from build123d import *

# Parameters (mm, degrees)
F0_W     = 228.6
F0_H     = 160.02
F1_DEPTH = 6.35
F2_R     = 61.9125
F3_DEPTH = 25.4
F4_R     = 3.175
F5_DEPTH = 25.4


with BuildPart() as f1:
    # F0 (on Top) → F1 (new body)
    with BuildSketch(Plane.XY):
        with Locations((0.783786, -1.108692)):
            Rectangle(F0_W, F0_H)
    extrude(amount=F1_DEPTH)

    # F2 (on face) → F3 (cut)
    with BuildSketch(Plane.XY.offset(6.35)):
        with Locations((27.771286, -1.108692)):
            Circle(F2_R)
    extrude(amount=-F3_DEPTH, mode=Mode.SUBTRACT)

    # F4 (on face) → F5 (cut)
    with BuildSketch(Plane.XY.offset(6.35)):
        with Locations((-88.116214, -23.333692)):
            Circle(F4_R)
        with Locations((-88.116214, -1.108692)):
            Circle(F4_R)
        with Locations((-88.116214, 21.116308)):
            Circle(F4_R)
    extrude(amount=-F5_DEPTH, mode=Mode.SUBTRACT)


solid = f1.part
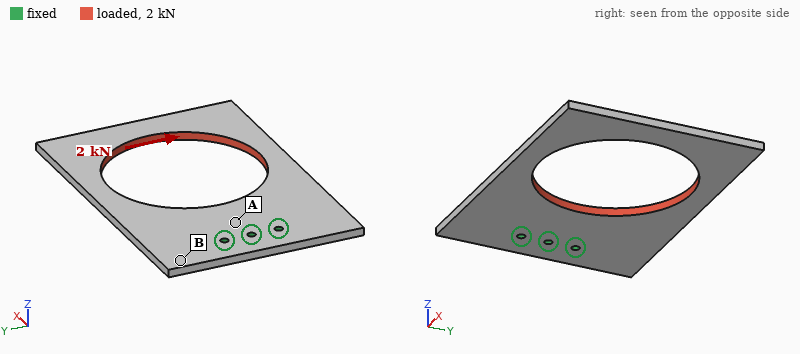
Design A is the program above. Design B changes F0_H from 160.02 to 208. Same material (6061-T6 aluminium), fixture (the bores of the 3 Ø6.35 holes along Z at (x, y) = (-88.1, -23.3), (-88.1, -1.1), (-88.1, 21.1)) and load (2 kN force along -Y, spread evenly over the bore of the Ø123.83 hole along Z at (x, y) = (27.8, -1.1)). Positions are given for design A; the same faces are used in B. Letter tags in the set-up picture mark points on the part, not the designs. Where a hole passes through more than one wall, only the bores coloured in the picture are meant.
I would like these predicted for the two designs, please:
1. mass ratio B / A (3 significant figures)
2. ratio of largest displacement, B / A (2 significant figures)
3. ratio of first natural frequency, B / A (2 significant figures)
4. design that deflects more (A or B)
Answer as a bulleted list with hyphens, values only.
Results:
- 1.45
- 0.74
- 0.98
- A
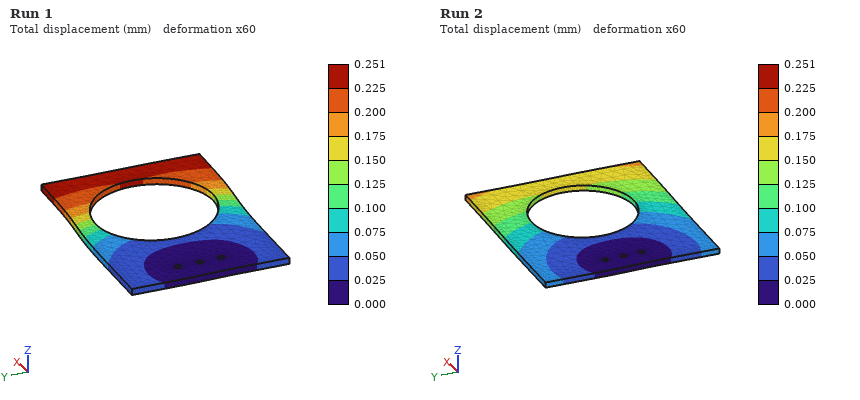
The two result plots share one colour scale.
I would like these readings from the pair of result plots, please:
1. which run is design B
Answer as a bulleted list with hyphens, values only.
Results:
- Run 2
